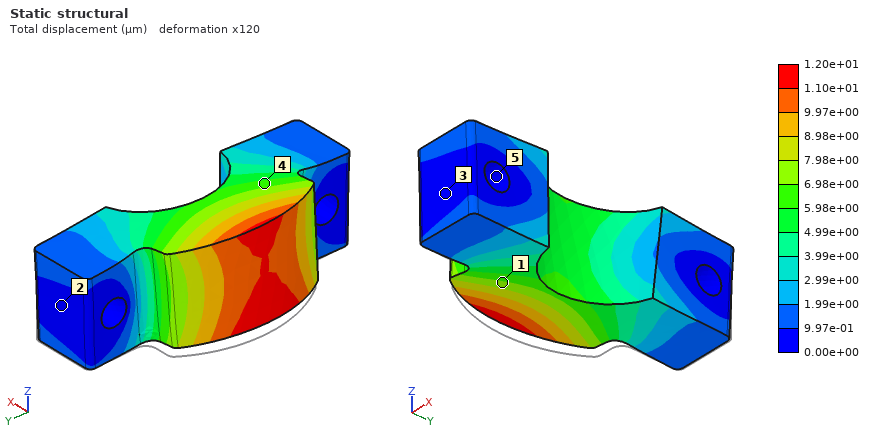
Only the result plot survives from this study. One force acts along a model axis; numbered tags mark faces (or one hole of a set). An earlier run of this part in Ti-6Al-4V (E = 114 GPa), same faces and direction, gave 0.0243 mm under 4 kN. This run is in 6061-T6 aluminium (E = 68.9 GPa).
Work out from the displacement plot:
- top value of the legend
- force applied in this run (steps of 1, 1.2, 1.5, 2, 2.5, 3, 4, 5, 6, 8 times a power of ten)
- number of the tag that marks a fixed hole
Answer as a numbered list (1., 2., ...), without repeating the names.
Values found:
1. 1.20e+01 µm
2. 1.2 kN
3. 5
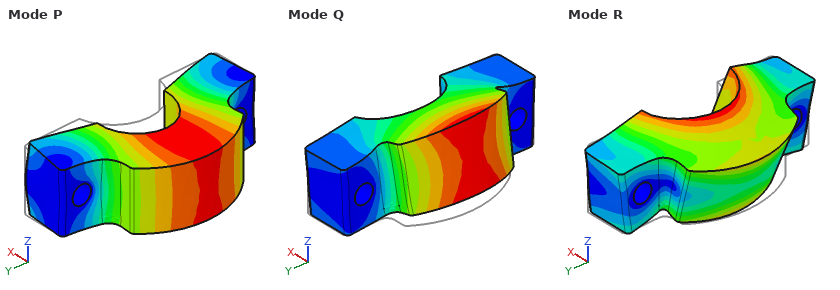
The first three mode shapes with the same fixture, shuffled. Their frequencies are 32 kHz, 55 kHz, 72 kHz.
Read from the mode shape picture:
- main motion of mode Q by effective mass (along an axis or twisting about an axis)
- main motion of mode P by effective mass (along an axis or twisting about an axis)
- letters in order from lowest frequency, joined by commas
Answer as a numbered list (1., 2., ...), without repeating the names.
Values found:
1. along Z
2. along X
3. Q, P, R
